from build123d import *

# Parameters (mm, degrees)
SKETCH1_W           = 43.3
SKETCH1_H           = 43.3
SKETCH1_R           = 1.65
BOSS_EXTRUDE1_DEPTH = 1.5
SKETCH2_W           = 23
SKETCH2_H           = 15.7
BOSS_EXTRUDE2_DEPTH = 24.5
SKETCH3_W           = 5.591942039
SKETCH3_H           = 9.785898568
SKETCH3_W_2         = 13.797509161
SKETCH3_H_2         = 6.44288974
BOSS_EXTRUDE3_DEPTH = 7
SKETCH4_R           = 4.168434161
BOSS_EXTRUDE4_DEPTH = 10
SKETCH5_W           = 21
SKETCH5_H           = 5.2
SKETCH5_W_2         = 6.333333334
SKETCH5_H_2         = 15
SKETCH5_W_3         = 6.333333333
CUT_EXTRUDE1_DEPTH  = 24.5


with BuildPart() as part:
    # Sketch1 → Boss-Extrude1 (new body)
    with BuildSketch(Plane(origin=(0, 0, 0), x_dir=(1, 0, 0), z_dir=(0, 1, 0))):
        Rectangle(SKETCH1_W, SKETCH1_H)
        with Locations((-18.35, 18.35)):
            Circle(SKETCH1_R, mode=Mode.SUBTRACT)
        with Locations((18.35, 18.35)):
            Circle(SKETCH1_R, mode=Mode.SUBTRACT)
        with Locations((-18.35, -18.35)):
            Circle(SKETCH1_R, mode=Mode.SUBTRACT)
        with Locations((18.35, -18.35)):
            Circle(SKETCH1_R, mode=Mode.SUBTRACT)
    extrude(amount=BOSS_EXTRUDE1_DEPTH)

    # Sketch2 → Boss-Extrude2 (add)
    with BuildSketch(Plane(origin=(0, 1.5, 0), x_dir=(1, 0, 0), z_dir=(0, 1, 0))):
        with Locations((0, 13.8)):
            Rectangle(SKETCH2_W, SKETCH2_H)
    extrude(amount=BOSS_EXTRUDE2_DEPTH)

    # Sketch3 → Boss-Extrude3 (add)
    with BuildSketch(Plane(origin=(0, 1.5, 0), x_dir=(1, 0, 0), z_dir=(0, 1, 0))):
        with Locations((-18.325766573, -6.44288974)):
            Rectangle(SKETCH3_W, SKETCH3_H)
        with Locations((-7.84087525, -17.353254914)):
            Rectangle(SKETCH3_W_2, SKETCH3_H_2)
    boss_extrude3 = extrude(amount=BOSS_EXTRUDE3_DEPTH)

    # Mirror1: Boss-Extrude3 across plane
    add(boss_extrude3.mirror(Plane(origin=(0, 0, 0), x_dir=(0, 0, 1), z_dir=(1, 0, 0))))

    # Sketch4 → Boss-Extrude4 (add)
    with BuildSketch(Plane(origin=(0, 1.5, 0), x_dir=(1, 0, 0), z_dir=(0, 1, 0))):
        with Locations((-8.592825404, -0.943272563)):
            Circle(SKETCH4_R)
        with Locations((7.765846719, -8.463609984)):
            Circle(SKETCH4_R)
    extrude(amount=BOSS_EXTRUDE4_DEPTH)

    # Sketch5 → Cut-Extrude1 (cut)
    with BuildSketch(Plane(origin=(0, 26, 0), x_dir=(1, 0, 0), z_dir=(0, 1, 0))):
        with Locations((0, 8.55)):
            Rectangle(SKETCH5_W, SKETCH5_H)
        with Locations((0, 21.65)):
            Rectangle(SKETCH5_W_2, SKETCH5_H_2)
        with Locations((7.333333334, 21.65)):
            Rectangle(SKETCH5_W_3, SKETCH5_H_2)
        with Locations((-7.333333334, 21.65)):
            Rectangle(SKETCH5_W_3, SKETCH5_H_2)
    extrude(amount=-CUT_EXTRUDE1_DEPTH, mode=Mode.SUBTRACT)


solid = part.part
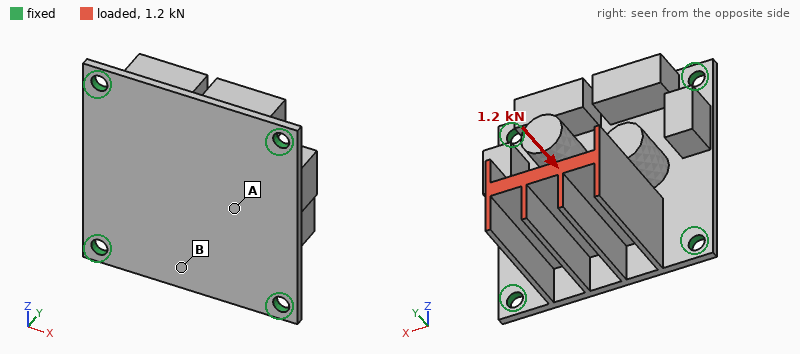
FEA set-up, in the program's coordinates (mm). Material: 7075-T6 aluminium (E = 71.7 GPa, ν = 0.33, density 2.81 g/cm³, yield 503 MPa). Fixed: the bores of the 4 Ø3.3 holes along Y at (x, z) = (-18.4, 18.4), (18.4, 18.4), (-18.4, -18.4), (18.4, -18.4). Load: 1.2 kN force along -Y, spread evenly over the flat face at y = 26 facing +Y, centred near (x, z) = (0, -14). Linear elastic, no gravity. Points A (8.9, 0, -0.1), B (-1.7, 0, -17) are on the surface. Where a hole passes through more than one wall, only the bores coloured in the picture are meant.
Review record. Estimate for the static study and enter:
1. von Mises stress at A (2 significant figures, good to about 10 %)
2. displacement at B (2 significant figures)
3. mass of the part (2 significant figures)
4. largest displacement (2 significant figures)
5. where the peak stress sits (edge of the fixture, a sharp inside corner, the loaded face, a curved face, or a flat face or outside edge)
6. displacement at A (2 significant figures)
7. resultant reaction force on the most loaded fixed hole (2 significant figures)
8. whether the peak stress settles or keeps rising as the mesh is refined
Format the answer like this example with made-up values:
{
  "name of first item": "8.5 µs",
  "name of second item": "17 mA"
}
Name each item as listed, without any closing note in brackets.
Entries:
{
  "von Mises stress at A": "46 MPa",
  "displacement at B": "0.093 mm",
  "mass of the part": "24 g",
  "largest displacement": "0.21 mm",
  "where the peak stress sits": "edge of the fixture",
  "displacement at A": "0.13 mm",
  "resultant reaction force on the most loaded fixed hole": "560 N",
  "whether the peak stress settles or keeps rising as the mesh is refined": "keeps rising"
}
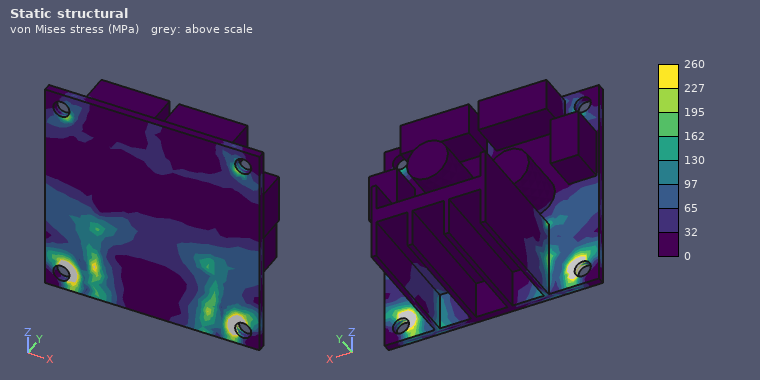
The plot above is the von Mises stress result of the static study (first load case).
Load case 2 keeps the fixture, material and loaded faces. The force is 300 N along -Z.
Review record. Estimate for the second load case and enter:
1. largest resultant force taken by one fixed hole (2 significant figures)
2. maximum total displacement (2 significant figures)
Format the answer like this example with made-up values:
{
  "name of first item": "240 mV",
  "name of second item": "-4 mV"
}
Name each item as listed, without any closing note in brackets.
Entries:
{
  "largest resultant force taken by one fixed hole": "140 N",
  "maximum total displacement": "0.48 mm"
}
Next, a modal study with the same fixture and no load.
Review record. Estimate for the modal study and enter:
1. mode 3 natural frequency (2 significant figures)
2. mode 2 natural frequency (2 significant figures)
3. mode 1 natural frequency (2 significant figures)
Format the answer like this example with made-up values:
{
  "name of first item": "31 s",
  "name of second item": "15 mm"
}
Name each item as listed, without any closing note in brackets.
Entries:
{
  "mode 3 natural frequency": "4400 Hz",
  "mode 2 natural frequency": "4300 Hz",
  "mode 1 natural frequency": "2200 Hz"
}
